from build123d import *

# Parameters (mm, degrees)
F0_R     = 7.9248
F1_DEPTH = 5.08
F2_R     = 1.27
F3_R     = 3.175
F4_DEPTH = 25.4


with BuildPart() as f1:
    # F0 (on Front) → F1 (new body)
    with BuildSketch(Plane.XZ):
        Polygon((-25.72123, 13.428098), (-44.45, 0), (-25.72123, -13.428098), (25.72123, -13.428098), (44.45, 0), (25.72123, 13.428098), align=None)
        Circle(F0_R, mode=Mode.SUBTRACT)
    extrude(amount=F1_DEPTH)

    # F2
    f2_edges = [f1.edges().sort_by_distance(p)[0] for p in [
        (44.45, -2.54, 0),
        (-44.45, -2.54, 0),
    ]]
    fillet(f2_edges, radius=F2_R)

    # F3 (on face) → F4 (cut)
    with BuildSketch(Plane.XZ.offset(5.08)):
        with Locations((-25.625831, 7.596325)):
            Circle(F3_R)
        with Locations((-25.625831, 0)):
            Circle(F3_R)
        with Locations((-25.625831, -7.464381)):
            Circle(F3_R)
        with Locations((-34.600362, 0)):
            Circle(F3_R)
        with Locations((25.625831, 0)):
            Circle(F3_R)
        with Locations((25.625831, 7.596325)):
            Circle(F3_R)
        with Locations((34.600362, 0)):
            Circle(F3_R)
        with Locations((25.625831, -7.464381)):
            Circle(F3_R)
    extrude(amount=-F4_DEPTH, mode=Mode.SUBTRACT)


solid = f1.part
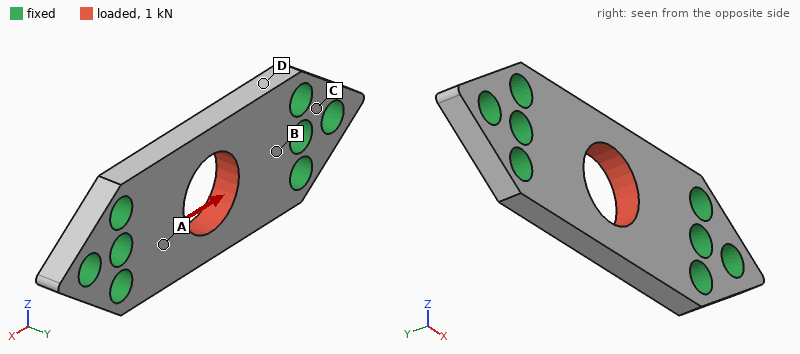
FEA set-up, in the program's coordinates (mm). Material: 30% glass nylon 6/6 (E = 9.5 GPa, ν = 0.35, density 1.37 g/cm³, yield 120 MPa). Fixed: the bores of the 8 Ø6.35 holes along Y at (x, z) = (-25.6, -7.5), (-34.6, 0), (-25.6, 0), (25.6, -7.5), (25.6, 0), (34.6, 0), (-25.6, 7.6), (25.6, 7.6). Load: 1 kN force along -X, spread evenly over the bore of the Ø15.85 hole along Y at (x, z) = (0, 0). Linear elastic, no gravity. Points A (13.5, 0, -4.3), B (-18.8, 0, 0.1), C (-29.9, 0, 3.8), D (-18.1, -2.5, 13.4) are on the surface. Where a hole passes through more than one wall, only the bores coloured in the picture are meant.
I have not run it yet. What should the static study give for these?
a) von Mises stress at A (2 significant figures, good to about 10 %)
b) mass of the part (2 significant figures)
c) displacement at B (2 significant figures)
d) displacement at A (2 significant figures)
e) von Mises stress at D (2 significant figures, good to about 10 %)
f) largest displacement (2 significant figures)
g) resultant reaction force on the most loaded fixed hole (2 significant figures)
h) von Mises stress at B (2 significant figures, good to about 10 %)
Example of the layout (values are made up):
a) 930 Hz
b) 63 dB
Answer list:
a) 4.4 MPa
b) 10.0 g
c) 1.5 µm
d) 3.9 µm
e) 2.5 MPa
f) 9.5 µm
g) 190 N
h) 3.8 MPa
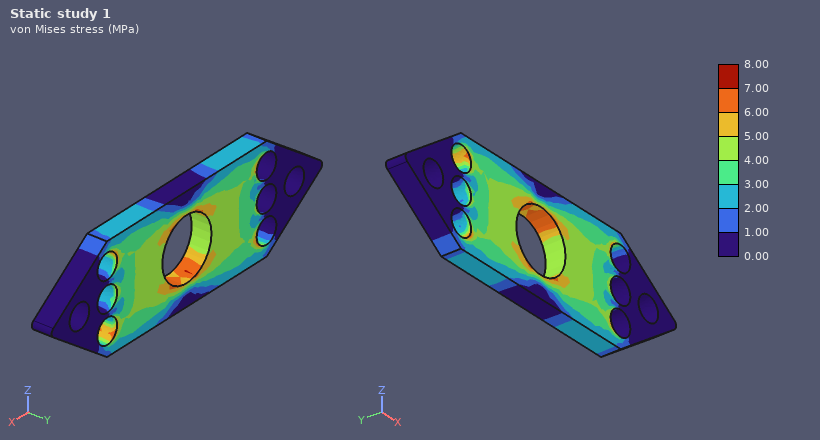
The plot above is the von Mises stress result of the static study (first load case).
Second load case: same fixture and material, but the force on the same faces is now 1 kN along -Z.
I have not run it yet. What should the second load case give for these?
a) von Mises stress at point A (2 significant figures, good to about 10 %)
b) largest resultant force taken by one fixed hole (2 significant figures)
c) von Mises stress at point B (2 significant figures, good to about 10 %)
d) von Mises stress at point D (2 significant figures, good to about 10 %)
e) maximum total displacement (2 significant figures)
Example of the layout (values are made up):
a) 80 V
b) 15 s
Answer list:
a) 8.8 MPa
b) 300 N
c) 9.1 MPa
d) 4.4 MPa
e) 36 µm
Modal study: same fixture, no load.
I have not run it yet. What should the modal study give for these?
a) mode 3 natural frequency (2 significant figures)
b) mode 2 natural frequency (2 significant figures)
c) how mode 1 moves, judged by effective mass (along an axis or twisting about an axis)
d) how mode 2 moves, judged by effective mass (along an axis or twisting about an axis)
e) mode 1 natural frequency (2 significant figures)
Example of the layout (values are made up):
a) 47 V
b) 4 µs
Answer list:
a) 14 kHz
b) 8200 Hz
c) along Y
d) twisting about X
e) 6700 Hz
